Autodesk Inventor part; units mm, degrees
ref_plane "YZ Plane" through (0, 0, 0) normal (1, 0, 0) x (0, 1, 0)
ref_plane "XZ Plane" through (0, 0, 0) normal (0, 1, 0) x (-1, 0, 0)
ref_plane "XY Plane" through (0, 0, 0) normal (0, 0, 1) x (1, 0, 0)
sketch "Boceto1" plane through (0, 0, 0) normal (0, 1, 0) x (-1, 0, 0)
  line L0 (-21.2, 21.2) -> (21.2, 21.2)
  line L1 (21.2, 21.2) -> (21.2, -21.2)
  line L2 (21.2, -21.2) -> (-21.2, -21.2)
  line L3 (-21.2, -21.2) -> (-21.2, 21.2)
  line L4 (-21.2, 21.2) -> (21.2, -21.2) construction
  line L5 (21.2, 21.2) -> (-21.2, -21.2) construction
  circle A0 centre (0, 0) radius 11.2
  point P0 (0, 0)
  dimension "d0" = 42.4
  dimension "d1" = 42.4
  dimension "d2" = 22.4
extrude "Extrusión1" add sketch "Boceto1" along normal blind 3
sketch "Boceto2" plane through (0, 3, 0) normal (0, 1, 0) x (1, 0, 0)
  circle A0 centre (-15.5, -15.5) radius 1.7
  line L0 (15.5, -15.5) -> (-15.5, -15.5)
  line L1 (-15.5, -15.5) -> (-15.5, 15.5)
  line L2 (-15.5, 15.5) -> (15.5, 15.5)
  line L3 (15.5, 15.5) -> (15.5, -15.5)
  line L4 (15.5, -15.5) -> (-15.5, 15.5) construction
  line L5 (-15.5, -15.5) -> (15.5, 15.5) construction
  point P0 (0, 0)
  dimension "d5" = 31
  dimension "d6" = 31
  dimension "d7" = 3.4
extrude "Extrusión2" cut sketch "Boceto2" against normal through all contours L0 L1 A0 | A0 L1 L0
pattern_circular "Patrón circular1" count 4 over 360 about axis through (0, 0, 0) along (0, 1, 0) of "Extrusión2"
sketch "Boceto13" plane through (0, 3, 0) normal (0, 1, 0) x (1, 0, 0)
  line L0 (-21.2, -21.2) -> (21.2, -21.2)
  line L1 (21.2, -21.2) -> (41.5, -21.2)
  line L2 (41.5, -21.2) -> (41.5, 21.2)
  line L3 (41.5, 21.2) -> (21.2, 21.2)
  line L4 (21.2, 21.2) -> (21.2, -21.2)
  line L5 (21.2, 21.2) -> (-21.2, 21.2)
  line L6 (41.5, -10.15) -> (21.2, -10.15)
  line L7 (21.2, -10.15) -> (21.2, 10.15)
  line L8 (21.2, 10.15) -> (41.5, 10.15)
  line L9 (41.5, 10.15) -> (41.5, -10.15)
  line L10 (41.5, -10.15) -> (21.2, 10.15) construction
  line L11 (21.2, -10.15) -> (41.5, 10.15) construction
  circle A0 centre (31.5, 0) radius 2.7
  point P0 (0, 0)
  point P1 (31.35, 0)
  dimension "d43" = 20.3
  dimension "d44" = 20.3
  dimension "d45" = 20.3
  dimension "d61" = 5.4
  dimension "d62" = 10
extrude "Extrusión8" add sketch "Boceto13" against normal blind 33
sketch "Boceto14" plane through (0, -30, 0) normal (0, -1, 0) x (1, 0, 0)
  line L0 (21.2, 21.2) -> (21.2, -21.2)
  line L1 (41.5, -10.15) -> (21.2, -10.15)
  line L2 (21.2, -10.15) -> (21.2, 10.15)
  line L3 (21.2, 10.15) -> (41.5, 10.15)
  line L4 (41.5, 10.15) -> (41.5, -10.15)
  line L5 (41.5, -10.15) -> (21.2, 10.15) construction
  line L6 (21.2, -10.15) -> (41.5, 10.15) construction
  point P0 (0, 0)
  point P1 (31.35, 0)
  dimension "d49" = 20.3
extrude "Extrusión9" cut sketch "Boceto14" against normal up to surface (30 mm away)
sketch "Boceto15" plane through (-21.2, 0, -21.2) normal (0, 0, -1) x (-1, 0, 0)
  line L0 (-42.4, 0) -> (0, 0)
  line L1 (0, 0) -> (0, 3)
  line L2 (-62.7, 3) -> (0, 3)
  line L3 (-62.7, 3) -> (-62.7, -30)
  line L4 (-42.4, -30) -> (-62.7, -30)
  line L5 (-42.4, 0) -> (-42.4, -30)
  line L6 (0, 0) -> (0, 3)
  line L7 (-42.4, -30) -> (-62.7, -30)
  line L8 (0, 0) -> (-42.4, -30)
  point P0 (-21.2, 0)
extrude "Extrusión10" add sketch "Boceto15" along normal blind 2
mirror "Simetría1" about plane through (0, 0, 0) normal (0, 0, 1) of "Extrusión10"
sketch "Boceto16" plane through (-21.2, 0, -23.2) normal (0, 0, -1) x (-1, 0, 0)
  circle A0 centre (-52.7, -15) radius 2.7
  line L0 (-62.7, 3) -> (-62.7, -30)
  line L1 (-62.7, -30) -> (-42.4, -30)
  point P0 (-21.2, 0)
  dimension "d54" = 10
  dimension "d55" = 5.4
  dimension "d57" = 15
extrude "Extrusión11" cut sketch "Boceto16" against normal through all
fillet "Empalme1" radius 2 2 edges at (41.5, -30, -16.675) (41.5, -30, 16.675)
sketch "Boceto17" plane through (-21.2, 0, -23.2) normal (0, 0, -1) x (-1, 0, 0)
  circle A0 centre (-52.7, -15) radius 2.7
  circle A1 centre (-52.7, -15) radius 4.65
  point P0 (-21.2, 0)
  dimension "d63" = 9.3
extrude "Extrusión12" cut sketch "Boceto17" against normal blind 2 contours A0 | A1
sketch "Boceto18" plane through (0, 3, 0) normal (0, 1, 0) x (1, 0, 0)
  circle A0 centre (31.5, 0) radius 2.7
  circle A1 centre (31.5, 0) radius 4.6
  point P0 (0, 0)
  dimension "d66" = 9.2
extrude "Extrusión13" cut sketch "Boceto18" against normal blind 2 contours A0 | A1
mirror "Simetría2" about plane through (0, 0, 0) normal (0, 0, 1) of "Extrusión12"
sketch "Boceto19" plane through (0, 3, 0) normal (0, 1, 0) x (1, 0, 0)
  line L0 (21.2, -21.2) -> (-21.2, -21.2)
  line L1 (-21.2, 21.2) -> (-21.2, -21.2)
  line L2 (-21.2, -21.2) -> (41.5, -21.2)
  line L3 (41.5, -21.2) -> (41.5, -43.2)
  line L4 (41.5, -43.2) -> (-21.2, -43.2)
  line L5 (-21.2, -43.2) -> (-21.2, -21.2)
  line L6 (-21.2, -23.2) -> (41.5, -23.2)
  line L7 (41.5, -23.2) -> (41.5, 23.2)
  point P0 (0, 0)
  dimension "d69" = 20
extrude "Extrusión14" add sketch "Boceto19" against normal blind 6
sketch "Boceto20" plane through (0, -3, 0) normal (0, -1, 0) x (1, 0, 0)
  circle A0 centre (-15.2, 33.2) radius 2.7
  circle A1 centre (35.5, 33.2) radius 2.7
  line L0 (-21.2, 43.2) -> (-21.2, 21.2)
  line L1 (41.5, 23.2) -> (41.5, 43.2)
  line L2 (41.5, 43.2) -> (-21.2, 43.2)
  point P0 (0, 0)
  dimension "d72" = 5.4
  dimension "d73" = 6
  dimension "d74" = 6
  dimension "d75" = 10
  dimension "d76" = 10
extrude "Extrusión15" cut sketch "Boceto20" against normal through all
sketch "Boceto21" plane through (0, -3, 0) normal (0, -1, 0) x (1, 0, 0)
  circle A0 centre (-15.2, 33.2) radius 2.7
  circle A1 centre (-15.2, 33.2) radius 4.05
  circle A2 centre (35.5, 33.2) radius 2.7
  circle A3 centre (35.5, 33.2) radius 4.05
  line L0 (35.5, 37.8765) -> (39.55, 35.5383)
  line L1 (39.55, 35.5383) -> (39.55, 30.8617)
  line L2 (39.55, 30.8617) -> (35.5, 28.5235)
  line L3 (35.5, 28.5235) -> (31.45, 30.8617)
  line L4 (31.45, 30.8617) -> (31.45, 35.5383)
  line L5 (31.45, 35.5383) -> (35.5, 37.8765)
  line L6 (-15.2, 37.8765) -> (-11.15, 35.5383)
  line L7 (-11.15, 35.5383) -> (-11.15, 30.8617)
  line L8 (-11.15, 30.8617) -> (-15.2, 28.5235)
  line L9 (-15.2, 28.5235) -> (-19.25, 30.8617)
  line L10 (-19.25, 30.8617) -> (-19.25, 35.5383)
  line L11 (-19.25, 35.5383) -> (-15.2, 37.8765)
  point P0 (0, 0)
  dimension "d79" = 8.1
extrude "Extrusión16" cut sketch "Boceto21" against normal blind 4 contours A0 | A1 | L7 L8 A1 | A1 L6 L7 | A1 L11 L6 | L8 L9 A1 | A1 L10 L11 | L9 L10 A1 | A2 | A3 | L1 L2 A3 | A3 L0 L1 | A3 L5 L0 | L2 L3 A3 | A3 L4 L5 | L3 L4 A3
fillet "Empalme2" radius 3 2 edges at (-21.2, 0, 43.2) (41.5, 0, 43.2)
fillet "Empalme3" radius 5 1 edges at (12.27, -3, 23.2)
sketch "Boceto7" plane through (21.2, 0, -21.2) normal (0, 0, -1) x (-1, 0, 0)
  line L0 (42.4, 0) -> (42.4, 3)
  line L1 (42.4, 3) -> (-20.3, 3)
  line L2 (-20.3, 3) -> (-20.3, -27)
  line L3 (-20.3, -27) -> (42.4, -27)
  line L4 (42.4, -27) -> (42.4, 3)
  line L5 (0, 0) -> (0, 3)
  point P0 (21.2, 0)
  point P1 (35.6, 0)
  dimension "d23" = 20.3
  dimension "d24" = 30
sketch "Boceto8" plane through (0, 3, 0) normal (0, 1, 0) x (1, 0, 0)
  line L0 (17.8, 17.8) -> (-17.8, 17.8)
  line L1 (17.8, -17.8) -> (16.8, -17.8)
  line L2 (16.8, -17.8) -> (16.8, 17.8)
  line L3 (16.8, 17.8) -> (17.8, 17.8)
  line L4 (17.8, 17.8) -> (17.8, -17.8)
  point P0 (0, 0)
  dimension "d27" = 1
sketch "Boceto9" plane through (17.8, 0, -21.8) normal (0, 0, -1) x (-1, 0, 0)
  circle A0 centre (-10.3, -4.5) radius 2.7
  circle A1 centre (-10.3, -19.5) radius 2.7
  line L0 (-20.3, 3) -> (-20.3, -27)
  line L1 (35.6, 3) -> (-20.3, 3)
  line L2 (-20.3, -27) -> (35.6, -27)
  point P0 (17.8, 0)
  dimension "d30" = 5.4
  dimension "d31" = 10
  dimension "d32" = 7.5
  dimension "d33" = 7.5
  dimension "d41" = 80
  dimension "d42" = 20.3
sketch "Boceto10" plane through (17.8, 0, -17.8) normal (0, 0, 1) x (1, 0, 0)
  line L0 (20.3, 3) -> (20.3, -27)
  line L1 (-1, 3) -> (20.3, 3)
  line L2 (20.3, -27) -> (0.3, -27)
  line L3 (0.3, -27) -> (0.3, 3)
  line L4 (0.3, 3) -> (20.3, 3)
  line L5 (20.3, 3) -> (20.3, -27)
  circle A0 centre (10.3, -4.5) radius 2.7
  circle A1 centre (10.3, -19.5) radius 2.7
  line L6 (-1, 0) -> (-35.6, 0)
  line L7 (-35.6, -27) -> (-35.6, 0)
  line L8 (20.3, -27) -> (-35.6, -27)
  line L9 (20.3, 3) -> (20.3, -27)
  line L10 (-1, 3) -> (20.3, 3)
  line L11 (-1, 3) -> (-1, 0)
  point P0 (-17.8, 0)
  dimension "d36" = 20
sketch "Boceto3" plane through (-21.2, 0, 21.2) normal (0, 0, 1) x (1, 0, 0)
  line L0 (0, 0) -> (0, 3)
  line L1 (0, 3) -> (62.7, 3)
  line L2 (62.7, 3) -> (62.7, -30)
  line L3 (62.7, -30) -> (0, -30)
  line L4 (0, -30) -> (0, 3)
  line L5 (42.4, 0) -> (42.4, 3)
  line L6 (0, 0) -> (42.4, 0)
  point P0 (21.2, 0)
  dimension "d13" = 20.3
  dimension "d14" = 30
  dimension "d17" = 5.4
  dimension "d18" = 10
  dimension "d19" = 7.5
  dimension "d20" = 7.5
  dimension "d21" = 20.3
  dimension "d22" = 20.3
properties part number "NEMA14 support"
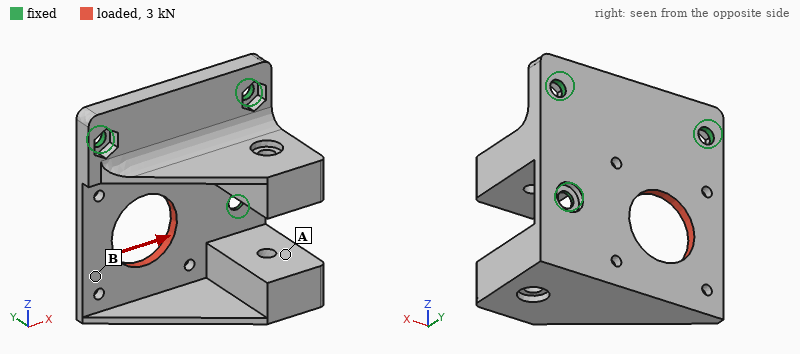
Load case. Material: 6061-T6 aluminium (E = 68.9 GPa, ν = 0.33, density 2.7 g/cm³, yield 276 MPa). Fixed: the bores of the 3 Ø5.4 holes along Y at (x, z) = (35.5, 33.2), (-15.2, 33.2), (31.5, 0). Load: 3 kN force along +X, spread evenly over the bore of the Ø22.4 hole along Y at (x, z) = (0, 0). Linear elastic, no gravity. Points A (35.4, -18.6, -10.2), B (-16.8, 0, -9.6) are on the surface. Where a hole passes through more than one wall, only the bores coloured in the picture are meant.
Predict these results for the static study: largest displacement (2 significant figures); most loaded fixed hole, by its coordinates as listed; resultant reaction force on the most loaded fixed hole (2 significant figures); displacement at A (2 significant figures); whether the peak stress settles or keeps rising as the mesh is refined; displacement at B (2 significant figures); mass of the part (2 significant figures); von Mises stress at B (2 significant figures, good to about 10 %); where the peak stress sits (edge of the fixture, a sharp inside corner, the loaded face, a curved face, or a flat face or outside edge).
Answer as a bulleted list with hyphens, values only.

- 97 µm
- (31.5, 0)
- 1.8 kN
- 18 µm
- keeps rising
- 67 µm
- 87 g
- 21 MPa
- edge of the fixture
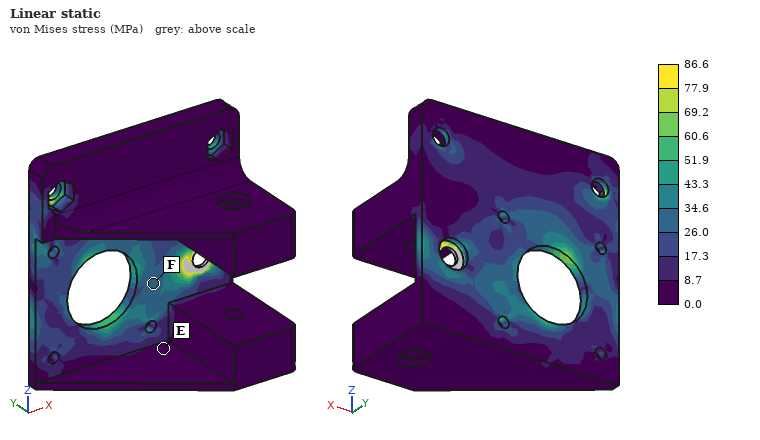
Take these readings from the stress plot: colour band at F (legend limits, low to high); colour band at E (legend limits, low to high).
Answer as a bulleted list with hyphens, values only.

- 26.0 to 34.6 MPa
- 0.0 to 8.7 MPa
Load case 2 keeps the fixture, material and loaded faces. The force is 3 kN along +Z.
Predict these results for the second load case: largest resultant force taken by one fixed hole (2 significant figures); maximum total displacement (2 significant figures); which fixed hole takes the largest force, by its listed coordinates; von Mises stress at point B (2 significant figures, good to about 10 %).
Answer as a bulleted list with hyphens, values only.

- 1.8 kN
- 32 µm
- (-15.2, 33.2)
- 8.6 MPa
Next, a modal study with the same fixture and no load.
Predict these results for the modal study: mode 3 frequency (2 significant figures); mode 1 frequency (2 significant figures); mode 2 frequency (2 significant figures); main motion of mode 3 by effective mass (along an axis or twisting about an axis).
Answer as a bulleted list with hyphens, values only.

- 4100 Hz
- 770 Hz
- 1300 Hz
- along Y
